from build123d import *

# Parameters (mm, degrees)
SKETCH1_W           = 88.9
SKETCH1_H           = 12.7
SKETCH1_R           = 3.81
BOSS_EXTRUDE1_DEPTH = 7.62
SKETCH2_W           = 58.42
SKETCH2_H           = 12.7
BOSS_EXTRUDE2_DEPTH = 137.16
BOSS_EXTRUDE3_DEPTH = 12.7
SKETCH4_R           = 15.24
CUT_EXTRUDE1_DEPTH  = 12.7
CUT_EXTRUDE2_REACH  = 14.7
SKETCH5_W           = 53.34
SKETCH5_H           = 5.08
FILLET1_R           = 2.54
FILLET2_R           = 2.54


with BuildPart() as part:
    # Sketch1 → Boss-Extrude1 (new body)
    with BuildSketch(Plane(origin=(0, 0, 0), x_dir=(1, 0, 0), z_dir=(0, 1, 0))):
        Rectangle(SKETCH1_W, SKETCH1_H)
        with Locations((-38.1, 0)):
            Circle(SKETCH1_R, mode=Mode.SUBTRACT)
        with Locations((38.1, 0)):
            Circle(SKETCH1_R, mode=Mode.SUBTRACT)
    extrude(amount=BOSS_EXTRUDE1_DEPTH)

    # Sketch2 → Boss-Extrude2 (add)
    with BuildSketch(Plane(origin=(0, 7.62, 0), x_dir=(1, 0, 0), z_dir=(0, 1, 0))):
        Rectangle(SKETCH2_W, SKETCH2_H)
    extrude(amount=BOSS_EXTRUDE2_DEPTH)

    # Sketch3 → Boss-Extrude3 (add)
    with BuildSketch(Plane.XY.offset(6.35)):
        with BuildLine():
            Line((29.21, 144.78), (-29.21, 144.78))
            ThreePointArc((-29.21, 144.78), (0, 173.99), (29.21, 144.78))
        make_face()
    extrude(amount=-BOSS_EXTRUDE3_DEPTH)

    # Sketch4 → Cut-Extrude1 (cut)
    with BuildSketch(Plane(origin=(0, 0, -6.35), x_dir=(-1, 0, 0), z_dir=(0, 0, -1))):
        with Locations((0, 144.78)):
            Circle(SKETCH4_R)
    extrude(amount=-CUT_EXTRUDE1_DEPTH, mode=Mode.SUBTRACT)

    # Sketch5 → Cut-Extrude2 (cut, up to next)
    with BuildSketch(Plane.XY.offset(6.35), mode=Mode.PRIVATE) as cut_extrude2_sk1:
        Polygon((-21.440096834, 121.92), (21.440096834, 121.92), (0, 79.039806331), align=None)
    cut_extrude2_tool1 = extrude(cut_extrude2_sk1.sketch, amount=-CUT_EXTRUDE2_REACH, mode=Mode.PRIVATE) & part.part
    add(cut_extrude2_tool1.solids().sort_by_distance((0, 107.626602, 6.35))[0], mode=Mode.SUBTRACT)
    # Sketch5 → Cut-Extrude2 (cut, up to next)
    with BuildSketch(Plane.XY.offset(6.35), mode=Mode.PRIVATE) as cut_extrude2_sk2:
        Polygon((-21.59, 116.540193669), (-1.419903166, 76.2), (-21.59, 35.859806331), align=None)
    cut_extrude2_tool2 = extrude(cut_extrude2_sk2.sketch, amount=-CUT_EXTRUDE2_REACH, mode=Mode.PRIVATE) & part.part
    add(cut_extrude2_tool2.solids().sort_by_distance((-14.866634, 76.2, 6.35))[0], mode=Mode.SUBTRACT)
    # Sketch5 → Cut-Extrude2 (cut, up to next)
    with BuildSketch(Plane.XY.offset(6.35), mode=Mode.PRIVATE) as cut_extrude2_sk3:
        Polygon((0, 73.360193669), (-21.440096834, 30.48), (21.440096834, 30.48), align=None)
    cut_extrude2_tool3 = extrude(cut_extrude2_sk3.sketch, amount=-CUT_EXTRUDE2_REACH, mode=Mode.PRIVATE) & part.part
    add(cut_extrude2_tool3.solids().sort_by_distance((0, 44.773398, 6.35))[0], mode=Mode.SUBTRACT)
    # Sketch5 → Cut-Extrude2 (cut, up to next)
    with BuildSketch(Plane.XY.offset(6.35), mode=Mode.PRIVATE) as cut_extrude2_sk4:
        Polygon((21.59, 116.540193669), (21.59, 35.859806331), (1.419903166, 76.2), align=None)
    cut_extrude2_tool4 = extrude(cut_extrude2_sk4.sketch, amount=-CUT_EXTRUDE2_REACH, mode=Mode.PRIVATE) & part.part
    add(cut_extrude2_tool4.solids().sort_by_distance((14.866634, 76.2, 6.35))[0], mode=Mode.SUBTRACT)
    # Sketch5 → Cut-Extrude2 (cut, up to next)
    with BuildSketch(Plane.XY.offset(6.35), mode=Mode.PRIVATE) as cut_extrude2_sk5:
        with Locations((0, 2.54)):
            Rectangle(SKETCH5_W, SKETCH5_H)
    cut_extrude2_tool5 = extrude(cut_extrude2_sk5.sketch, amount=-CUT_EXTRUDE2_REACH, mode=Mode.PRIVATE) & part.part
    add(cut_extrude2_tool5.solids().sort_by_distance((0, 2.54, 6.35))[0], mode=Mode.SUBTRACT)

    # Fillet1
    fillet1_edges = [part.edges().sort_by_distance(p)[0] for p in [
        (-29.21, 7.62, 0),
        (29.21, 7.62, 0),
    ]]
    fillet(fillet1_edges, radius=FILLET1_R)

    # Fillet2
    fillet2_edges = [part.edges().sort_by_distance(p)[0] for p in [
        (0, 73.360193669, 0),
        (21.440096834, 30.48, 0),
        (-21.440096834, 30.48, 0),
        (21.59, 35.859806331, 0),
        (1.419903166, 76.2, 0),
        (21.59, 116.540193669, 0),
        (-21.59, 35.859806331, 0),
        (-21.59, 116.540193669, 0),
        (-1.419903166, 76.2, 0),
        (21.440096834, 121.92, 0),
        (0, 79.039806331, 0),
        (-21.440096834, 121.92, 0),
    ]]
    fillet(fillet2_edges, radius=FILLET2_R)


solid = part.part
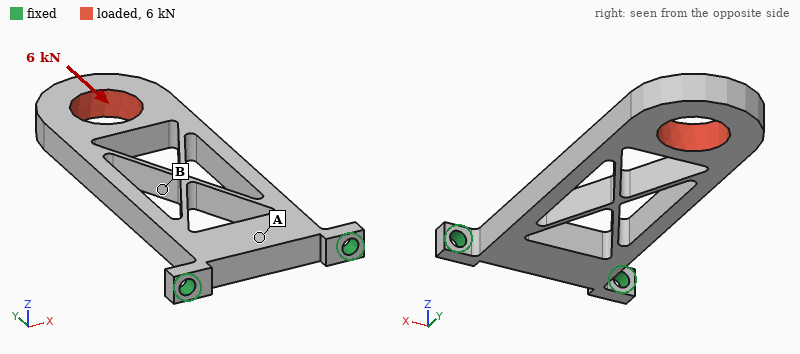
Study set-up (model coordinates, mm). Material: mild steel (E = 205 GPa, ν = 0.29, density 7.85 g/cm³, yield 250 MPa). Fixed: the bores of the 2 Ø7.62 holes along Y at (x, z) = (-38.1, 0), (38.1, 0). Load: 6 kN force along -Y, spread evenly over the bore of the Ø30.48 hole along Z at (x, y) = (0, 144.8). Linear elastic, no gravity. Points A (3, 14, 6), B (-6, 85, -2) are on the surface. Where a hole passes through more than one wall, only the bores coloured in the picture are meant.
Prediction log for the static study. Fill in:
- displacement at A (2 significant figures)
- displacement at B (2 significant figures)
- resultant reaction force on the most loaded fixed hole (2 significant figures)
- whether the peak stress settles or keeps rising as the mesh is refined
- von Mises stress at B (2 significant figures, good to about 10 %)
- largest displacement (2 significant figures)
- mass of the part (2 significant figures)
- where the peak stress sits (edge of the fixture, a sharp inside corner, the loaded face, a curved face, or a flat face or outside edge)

7.1 µm
16 µm
3.4 kN
keeps rising
25 MPa
26 µm
560 g
edge of the fixture
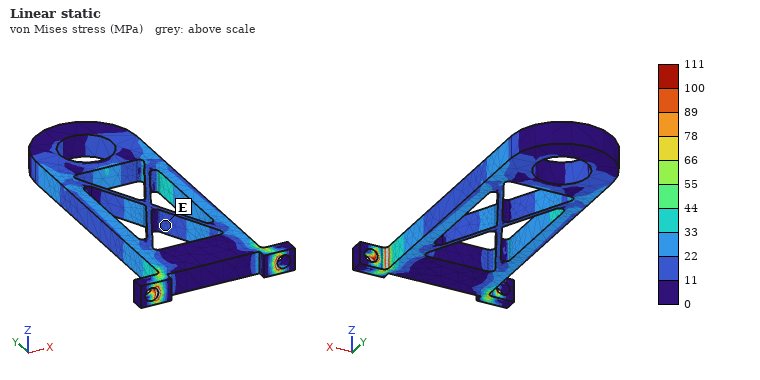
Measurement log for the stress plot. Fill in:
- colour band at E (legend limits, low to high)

11 to 22 MPa
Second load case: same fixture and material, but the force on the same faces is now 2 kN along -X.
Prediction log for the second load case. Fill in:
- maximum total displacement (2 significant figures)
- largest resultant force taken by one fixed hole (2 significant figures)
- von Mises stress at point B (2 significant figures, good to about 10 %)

0.20 mm
4.8 kN
60 MPa
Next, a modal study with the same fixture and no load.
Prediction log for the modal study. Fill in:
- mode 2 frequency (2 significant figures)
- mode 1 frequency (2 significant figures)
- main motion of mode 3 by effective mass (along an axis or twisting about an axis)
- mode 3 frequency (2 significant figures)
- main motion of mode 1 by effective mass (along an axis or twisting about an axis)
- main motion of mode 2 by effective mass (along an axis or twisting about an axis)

1100 Hz
220 Hz
twisting about Y
1200 Hz
along Z
along X
